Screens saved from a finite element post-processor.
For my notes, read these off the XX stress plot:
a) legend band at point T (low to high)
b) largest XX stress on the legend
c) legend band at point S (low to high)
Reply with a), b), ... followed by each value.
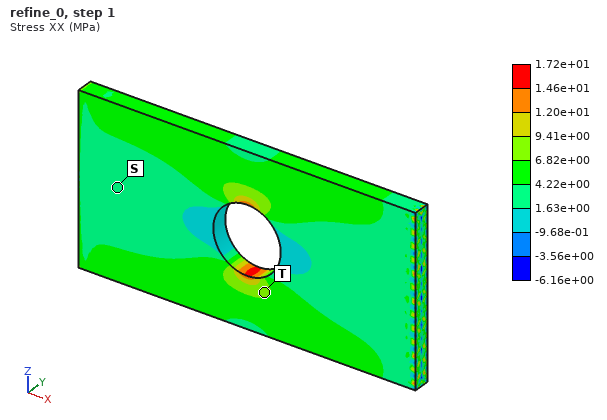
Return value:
a) 6.82e+00 to 9.41e+00 MPa
b) 1.72e+01 MPa
c) 1.63e+00 to 4.22e+00 MPa
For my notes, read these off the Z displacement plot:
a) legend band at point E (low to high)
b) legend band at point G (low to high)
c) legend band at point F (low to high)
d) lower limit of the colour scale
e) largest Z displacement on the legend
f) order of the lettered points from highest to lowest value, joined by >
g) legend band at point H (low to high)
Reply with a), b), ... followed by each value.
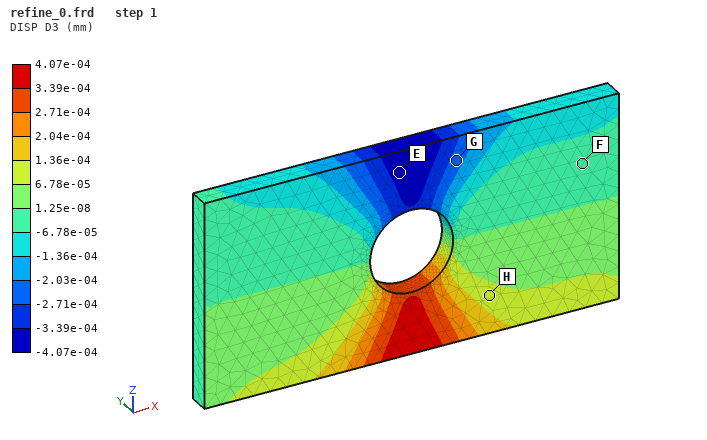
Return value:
a) -4.07e-04 to -3.39e-04 mm
b) -2.71e-04 to -2.03e-04 mm
c) -6.78e-05 to 1.25e-08 mm
d) -4.07e-04 mm
e) 4.07e-04 mm
f) H > F > G > E
g) 6.78e-05 to 1.36e-04 mm
